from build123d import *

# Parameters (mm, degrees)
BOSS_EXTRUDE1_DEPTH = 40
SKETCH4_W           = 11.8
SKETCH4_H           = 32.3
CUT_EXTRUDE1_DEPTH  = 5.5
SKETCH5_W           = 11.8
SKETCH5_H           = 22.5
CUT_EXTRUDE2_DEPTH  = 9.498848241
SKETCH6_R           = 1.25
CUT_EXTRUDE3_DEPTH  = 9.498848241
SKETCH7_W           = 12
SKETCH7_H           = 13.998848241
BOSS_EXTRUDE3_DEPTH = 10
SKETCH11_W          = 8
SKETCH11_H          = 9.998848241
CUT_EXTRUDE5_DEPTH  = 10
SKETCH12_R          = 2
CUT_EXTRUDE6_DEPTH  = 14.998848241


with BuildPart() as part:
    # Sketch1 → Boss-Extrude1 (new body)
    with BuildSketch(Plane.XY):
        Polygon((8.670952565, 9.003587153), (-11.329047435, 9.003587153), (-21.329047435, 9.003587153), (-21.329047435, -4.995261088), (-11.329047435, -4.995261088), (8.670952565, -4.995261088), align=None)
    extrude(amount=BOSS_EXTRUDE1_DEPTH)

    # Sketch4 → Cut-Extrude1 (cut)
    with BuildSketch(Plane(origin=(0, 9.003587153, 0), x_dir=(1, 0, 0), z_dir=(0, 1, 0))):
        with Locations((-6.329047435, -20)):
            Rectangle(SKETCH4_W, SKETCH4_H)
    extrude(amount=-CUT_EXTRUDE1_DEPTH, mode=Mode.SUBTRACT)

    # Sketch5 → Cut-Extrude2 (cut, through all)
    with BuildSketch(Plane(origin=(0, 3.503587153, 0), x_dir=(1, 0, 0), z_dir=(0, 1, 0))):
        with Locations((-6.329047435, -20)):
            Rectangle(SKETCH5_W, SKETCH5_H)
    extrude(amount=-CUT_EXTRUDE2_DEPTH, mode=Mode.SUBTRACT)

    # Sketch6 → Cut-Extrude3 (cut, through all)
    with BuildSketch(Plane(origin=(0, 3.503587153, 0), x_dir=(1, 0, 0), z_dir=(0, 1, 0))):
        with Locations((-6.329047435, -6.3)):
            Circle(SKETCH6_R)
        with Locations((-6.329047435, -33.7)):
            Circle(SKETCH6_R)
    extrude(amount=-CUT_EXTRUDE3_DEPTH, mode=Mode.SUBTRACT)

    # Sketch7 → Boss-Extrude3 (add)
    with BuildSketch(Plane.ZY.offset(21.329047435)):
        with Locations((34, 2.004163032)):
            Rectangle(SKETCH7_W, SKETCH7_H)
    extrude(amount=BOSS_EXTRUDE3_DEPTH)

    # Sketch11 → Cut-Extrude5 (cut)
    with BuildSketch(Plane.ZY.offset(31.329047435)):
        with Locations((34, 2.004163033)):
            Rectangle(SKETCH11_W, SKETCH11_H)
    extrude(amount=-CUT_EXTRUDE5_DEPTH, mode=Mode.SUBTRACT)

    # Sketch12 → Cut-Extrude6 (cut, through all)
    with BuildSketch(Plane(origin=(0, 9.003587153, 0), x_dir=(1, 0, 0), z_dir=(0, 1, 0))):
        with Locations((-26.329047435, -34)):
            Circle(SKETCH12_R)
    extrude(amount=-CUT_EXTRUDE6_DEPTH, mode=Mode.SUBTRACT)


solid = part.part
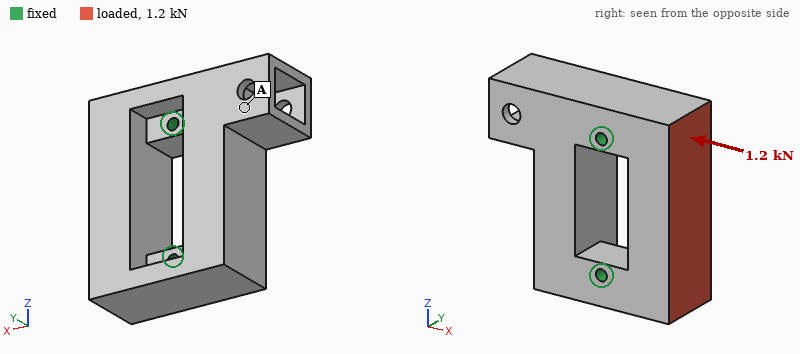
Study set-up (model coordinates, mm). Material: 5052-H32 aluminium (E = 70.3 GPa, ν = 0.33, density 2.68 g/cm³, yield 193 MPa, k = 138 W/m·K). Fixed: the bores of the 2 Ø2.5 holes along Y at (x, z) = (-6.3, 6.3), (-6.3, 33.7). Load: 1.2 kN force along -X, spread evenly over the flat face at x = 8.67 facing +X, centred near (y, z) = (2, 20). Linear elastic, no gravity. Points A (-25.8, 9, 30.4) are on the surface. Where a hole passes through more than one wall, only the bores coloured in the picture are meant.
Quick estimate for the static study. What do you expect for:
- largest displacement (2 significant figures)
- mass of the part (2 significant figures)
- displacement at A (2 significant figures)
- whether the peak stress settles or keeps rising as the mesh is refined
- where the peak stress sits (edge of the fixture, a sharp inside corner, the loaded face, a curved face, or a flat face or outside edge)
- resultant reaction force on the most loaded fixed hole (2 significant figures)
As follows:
7.8 µm
35 g
3.0 µm
keeps rising
edge of the fixture
630 N
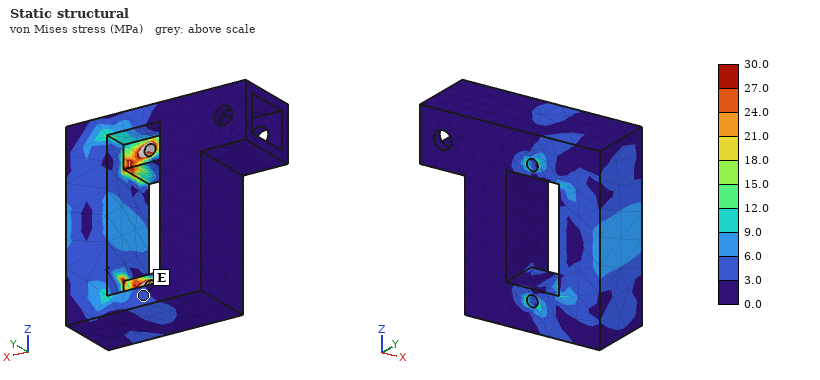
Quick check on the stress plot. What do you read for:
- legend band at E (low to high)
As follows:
3.0 to 6.0 MPa
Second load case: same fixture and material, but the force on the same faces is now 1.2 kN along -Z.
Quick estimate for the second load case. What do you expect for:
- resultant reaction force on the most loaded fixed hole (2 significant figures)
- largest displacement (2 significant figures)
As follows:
790 N
10 µm
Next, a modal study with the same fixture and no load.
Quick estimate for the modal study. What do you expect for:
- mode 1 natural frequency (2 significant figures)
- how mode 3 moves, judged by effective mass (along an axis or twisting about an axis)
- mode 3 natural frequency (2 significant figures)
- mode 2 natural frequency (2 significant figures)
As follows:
9500 Hz
along Y
15 kHz
14 kHz
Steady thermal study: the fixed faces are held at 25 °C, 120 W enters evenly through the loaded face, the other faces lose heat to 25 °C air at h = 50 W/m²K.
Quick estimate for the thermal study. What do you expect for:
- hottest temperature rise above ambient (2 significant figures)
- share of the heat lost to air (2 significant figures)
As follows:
65 K
4.1 %
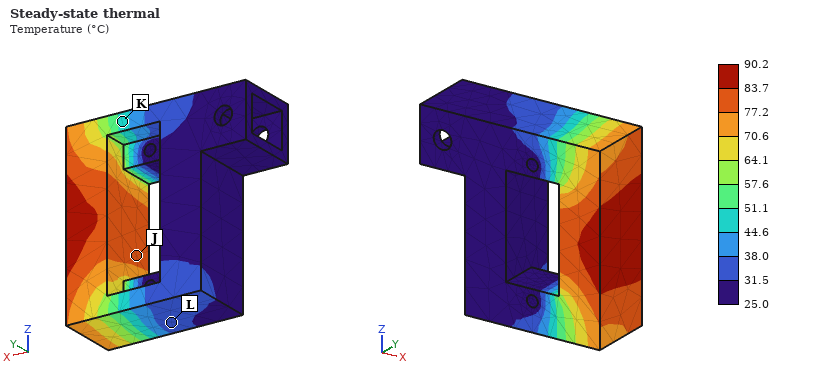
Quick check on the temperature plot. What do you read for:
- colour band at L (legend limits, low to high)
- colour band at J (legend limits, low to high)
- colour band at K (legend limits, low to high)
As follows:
31.5 to 38.0 °C
77.2 to 83.7 °C
44.6 to 51.1 °C
